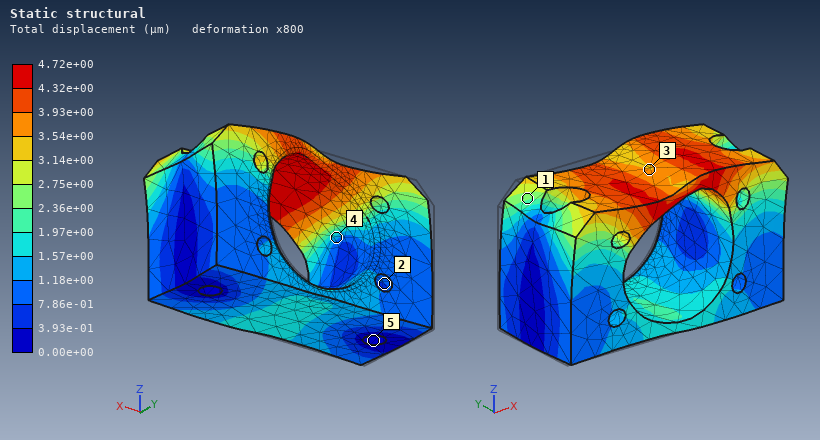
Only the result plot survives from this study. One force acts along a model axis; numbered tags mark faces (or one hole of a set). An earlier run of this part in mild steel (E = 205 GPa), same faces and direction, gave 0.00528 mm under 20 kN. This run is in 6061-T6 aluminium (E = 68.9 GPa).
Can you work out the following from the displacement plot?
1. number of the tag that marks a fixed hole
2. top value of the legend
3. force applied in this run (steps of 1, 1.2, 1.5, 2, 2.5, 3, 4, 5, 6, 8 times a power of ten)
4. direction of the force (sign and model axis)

5
4.72e+00 µm
6 kN
+X
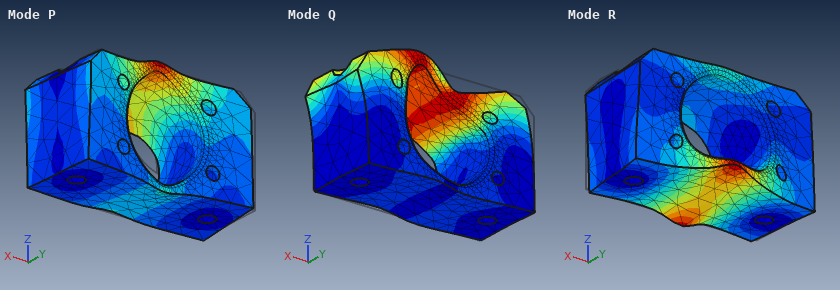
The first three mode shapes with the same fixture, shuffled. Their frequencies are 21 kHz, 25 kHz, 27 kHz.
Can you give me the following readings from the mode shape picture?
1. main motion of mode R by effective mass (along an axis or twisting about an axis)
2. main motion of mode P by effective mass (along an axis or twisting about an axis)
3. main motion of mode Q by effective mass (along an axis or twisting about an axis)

twisting about X
along Y
along X
